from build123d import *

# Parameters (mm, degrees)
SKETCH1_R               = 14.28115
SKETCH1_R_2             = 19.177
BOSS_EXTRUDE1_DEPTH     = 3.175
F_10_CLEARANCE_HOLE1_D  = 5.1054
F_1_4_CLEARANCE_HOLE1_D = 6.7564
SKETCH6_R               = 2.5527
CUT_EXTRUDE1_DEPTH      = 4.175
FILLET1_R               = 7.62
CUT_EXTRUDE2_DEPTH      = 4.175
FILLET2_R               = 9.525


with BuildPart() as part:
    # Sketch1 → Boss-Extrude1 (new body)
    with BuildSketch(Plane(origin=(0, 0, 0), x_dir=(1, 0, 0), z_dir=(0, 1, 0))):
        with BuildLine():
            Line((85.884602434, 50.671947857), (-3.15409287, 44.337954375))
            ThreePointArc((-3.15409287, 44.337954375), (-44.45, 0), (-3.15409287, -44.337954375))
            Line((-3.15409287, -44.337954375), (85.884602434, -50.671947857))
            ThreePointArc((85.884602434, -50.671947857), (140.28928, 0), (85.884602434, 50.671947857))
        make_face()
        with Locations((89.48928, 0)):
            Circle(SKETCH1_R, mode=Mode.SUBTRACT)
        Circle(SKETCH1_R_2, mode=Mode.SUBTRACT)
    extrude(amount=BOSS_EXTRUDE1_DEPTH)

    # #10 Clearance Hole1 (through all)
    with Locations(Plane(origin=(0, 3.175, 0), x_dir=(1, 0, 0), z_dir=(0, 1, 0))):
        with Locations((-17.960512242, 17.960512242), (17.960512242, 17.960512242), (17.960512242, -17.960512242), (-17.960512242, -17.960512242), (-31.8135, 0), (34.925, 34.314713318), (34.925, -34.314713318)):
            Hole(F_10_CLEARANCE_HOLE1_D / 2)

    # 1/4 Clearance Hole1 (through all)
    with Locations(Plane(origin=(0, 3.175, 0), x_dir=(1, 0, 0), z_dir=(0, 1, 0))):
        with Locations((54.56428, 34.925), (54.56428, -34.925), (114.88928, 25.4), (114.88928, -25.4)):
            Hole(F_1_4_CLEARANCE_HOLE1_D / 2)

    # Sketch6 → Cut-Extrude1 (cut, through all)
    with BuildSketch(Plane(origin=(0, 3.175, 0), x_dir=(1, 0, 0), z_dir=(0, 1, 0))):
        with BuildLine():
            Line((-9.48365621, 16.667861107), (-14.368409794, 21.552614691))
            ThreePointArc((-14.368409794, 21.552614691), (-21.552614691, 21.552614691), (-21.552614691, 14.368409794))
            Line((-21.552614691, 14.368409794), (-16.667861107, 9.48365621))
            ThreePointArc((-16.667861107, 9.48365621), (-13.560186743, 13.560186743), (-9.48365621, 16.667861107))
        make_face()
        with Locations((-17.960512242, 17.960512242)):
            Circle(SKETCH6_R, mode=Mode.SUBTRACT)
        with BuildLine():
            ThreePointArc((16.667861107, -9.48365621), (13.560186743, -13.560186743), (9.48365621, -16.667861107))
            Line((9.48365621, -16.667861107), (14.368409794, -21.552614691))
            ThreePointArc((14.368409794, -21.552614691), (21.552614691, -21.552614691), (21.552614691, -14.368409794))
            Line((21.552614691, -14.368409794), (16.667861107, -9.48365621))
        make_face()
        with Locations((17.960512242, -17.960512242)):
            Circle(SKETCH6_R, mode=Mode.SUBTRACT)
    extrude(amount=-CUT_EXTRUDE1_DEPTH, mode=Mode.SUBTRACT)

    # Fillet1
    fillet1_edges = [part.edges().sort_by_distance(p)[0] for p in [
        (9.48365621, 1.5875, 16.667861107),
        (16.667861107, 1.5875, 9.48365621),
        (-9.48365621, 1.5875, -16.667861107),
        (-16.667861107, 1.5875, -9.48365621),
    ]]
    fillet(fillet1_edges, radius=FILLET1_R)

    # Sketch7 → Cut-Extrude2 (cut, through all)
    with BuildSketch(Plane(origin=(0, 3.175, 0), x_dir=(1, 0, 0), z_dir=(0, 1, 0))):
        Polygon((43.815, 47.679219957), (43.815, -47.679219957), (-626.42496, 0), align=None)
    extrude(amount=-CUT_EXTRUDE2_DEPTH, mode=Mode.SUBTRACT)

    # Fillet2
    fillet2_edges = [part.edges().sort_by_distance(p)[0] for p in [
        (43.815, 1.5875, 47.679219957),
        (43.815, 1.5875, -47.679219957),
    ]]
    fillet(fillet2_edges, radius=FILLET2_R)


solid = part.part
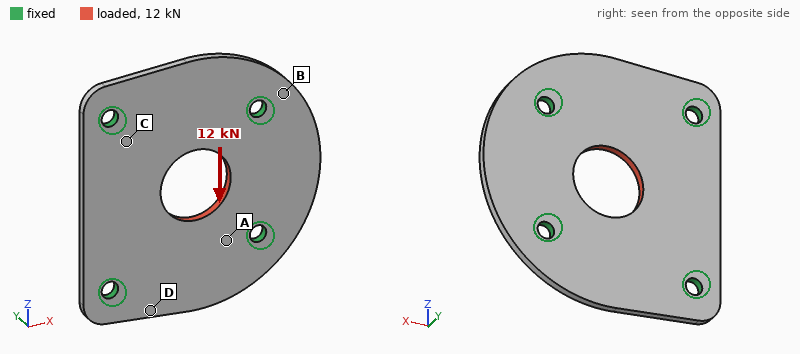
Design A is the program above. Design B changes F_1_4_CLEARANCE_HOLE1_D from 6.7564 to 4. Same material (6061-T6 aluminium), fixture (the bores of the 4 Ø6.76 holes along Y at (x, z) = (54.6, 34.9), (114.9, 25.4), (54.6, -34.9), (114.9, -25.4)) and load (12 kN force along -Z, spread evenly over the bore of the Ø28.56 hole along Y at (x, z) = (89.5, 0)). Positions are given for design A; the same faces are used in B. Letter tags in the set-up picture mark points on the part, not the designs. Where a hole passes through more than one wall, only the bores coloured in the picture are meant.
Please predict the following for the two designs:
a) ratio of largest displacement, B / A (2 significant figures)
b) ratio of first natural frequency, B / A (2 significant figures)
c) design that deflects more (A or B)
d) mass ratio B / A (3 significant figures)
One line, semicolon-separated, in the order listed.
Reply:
1.1; 0.89; B; 1.01
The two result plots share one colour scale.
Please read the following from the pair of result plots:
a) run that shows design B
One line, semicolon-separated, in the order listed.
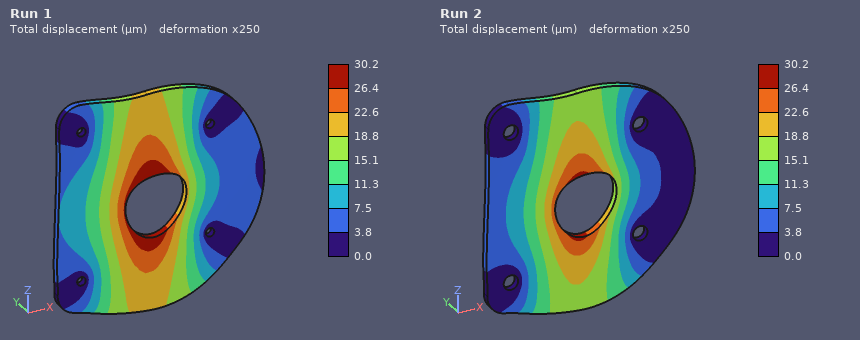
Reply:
Run 1
